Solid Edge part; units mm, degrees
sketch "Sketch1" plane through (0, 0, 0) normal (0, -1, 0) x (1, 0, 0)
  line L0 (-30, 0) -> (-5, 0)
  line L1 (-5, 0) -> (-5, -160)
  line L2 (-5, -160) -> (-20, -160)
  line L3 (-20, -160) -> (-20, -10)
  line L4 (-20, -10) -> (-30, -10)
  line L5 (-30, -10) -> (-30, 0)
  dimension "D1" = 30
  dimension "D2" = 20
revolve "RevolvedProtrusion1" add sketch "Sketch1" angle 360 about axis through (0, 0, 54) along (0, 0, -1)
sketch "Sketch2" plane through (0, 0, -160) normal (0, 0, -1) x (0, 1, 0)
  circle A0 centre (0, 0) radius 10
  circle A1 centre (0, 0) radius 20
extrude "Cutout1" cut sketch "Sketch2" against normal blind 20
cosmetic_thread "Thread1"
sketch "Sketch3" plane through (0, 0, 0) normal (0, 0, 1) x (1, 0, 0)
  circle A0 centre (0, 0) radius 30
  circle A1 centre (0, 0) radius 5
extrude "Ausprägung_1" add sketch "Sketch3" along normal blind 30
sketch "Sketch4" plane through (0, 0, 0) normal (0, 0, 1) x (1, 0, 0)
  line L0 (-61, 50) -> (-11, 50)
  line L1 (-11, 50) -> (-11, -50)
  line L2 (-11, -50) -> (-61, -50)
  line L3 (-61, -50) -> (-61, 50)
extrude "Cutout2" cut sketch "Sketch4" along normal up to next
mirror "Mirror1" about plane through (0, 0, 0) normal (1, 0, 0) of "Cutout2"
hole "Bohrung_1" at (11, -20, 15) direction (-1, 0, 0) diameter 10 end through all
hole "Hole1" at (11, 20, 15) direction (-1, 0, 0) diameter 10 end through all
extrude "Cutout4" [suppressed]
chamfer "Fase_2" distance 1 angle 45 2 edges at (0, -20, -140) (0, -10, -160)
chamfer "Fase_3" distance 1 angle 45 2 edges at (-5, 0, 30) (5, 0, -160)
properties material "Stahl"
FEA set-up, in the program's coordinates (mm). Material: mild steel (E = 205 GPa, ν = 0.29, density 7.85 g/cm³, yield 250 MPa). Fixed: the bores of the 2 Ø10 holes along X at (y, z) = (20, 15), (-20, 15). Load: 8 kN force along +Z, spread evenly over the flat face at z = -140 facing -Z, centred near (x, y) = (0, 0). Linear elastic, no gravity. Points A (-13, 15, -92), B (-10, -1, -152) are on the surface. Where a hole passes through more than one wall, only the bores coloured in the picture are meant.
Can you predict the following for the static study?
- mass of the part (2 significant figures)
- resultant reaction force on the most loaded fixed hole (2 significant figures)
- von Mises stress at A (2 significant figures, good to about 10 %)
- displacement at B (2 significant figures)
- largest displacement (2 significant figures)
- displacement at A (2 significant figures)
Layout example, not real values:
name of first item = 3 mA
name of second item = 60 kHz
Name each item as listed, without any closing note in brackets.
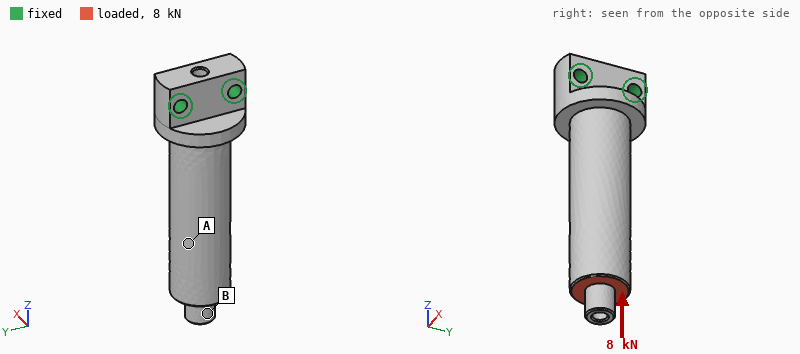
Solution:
mass of the part = 1.7 kg
resultant reaction force on the most loaded fixed hole = 4.1 kN
von Mises stress at A = 6.8 MPa
displacement at B = 5.2 µm
largest displacement = 5.4 µm
displacement at A = 3.8 µm
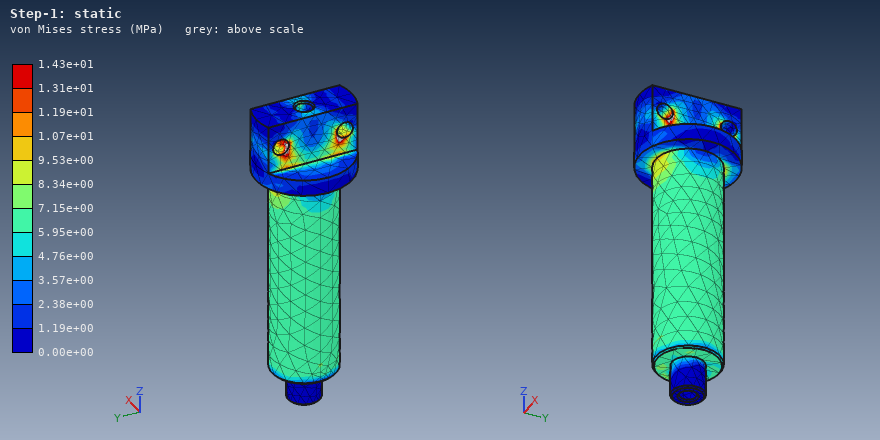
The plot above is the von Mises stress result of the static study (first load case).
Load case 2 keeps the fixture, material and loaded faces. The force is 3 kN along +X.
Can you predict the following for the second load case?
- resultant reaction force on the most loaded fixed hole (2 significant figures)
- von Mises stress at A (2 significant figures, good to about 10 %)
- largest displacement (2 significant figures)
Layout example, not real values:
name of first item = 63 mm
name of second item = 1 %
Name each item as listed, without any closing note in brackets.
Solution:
resultant reaction force on the most loaded fixed hole = 1.5 kN
von Mises stress at A = 16 MPa
largest displacement = 0.27 mm
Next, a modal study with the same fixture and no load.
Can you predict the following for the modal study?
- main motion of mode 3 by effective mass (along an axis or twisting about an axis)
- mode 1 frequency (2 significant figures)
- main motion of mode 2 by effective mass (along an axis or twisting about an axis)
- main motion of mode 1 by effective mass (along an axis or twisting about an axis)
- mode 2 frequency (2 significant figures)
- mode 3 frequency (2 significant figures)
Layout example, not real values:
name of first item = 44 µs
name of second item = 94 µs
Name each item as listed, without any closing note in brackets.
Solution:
main motion of mode 3 by effective mass = twisting about Z
mode 1 frequency = 860 Hz
main motion of mode 2 by effective mass = along Y
main motion of mode 1 by effective mass = along X
mode 2 frequency = 1300 Hz
mode 3 frequency = 5300 Hz
